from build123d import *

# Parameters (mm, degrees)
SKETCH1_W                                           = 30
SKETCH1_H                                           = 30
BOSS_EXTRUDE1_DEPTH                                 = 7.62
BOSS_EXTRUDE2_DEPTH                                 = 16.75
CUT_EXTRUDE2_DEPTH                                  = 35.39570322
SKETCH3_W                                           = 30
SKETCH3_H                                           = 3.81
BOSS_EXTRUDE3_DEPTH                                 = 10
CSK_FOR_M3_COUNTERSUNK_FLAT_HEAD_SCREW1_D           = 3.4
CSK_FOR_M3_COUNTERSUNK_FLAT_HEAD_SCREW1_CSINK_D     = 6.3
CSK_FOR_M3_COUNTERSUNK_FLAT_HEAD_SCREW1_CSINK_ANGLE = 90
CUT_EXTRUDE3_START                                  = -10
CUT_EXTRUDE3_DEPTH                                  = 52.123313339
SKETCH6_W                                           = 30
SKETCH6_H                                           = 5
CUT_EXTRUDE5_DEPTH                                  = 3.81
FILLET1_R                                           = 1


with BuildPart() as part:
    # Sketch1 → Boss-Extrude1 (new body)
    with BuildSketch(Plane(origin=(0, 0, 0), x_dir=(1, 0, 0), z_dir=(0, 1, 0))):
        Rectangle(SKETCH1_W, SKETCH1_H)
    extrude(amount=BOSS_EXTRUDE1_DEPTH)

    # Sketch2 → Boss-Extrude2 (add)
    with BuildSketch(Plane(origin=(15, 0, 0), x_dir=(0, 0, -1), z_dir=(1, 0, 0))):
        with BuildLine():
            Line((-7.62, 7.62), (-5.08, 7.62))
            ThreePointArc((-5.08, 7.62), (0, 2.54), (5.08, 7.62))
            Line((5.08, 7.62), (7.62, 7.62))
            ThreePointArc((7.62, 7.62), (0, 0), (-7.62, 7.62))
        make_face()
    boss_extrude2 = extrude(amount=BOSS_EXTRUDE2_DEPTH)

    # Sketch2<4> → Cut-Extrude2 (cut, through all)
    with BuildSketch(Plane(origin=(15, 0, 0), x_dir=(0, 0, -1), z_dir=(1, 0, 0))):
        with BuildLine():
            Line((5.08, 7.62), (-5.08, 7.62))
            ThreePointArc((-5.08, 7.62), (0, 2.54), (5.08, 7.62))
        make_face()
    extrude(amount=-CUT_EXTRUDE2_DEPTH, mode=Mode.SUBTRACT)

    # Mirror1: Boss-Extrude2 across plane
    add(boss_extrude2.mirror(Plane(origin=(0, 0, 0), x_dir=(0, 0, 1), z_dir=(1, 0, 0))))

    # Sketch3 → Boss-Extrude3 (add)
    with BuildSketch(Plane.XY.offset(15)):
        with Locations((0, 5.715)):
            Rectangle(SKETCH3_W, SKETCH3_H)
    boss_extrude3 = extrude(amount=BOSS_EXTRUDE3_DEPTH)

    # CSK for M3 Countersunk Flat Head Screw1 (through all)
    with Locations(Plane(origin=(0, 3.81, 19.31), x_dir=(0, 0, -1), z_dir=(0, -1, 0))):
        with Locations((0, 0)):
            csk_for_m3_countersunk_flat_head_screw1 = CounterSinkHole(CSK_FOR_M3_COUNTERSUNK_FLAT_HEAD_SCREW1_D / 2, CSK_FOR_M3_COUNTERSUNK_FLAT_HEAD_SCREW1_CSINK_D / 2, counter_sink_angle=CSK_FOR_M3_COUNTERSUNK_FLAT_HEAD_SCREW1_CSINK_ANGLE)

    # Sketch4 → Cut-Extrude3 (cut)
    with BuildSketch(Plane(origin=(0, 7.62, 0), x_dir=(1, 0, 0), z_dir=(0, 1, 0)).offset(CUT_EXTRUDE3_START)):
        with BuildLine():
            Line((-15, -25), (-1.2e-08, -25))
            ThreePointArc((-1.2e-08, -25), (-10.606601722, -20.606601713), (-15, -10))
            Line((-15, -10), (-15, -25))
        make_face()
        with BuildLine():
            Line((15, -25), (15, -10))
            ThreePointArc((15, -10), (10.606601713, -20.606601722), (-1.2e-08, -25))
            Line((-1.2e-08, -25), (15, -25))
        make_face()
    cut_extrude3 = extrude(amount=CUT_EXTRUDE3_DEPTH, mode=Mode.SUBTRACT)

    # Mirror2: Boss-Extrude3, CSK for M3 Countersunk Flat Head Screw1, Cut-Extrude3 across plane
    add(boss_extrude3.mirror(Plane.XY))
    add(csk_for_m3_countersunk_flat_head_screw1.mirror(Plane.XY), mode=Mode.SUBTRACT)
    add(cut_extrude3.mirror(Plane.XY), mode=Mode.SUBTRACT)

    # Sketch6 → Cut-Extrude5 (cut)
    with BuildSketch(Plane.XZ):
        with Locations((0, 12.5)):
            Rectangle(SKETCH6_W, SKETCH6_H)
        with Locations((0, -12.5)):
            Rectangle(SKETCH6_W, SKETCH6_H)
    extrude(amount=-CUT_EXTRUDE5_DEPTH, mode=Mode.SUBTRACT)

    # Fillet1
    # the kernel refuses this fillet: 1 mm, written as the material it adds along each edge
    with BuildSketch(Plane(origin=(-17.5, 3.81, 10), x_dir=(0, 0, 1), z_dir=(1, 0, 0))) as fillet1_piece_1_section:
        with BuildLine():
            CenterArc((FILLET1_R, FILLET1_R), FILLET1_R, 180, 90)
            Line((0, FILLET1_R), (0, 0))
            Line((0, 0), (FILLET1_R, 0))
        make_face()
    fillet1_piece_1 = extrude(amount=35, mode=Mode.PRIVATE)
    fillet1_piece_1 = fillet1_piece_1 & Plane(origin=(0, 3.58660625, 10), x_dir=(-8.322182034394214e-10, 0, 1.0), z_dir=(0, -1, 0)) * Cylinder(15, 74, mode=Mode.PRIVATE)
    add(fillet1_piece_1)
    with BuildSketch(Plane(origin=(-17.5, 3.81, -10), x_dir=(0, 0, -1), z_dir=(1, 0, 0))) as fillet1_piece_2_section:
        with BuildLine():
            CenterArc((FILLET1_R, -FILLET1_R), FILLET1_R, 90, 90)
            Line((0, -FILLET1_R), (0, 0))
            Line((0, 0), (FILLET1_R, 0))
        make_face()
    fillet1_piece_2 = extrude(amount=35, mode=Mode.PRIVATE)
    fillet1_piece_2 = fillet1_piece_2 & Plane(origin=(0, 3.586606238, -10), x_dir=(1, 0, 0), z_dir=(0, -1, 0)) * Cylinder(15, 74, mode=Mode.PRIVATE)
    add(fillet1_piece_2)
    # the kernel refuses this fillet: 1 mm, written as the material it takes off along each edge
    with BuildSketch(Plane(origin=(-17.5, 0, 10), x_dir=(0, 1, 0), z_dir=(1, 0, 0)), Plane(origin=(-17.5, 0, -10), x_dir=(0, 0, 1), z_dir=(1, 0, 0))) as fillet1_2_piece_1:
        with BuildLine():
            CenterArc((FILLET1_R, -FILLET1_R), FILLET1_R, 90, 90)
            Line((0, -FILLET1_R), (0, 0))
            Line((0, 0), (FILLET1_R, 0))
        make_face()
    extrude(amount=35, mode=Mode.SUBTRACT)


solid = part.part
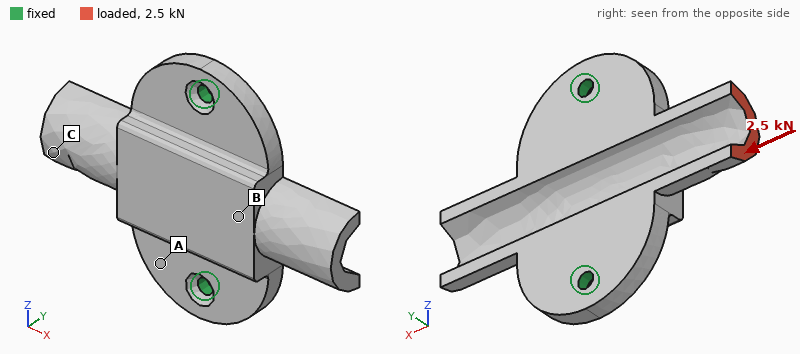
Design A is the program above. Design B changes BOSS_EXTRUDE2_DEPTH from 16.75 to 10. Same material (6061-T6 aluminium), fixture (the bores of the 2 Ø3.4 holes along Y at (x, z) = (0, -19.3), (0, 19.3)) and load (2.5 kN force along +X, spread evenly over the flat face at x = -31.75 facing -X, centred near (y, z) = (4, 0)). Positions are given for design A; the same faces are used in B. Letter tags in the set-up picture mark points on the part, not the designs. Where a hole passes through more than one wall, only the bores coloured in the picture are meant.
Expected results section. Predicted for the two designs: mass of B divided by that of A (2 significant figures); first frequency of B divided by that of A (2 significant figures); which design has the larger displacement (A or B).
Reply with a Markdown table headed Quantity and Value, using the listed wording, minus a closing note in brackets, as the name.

| Quantity | Value |
|---|---|
| mass of B divided by that of A | 0.91 |
| first frequency of B divided by that of A | 1.3 |
| which design has the larger displacement | A |
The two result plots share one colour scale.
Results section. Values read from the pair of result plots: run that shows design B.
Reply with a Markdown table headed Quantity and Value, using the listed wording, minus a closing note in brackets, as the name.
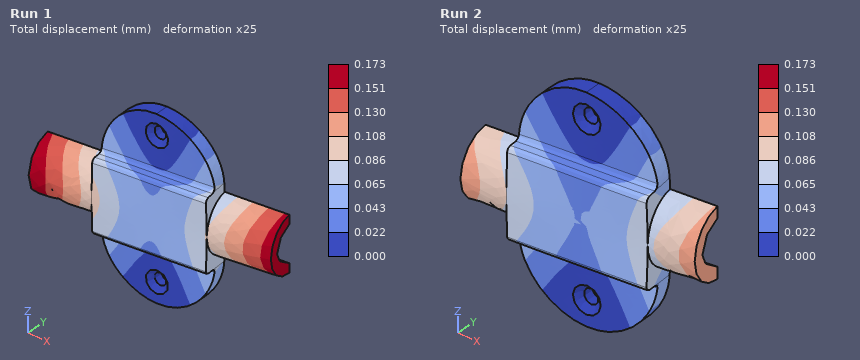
| Quantity | Value |
|---|---|
| run that shows design B | Run 2 |
